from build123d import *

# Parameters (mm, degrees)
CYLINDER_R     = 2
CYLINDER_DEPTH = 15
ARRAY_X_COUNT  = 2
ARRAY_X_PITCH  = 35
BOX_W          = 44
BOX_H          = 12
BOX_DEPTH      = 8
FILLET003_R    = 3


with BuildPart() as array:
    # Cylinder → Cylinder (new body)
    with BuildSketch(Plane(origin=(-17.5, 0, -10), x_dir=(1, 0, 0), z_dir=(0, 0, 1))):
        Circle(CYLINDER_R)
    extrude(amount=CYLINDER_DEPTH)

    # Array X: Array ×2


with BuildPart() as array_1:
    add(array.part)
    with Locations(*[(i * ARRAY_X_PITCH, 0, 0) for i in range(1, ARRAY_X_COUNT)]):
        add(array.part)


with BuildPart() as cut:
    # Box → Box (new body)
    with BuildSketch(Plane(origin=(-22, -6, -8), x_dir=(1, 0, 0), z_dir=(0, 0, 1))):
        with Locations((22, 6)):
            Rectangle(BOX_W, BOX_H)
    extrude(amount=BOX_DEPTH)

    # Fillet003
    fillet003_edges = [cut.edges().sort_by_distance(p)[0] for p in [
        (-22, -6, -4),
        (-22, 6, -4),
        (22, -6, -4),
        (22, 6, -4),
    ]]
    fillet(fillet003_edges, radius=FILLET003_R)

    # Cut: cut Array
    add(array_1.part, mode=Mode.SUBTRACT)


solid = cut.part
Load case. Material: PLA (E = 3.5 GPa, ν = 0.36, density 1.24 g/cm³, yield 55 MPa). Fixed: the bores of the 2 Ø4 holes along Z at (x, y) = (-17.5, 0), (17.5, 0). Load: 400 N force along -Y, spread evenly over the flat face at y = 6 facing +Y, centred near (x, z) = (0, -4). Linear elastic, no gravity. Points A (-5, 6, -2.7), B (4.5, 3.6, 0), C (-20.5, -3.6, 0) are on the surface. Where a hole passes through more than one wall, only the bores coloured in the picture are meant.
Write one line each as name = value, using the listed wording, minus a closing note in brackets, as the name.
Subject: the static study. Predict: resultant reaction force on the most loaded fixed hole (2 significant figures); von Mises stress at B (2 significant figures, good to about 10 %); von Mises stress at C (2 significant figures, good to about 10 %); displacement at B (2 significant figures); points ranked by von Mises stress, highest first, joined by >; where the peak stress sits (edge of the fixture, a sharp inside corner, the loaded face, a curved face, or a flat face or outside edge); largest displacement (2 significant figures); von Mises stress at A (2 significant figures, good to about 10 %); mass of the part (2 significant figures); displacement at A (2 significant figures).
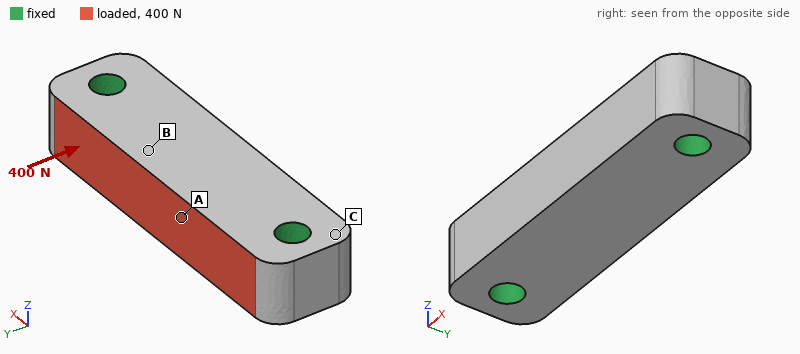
resultant reaction force on the most loaded fixed hole = 200 N
von Mises stress at B = 2.2 MPa
von Mises stress at C = 1.1 MPa
displacement at B = 29 µm
points ranked by von Mises stress, highest first, joined by > = A > B > C
where the peak stress sits = edge of the fixture
largest displacement = 32 µm
von Mises stress at A = 3.6 MPa
mass of the part = 4.9 g
displacement at A = 29 µm
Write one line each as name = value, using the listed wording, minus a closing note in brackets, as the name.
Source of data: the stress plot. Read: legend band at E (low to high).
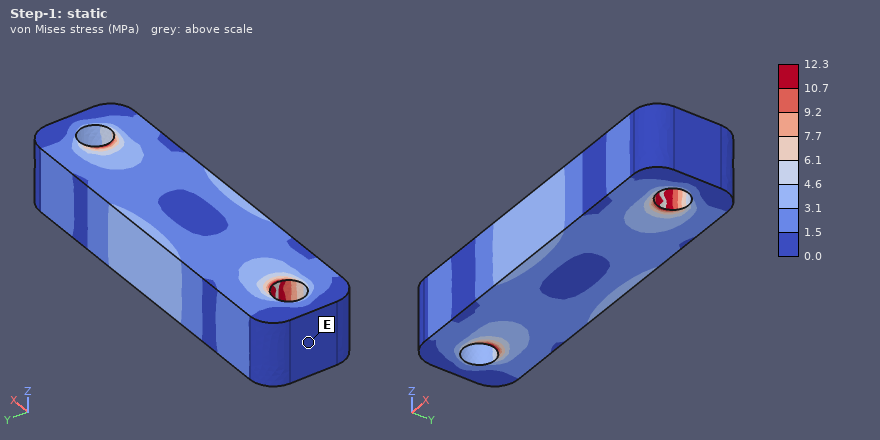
legend band at E = 0.0 to 1.5 MPa
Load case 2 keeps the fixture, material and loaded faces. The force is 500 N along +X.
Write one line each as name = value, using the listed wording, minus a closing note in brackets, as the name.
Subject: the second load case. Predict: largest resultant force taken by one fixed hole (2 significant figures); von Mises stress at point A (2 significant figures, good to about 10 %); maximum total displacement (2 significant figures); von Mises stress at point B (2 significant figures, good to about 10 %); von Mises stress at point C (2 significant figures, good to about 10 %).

largest resultant force taken by one fixed hole = 260 N
von Mises stress at point A = 3.0 MPa
maximum total displacement = 12 µm
von Mises stress at point B = 2.3 MPa
von Mises stress at point C = 0.92 MPa
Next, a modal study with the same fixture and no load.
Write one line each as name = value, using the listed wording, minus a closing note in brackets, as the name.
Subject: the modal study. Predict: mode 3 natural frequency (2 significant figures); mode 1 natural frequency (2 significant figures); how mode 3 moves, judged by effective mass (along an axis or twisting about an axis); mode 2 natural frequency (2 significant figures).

mode 3 natural frequency = 13 kHz
mode 1 natural frequency = 9000 Hz
how mode 3 moves, judged by effective mass = twisting about X
mode 2 natural frequency = 9300 Hz
